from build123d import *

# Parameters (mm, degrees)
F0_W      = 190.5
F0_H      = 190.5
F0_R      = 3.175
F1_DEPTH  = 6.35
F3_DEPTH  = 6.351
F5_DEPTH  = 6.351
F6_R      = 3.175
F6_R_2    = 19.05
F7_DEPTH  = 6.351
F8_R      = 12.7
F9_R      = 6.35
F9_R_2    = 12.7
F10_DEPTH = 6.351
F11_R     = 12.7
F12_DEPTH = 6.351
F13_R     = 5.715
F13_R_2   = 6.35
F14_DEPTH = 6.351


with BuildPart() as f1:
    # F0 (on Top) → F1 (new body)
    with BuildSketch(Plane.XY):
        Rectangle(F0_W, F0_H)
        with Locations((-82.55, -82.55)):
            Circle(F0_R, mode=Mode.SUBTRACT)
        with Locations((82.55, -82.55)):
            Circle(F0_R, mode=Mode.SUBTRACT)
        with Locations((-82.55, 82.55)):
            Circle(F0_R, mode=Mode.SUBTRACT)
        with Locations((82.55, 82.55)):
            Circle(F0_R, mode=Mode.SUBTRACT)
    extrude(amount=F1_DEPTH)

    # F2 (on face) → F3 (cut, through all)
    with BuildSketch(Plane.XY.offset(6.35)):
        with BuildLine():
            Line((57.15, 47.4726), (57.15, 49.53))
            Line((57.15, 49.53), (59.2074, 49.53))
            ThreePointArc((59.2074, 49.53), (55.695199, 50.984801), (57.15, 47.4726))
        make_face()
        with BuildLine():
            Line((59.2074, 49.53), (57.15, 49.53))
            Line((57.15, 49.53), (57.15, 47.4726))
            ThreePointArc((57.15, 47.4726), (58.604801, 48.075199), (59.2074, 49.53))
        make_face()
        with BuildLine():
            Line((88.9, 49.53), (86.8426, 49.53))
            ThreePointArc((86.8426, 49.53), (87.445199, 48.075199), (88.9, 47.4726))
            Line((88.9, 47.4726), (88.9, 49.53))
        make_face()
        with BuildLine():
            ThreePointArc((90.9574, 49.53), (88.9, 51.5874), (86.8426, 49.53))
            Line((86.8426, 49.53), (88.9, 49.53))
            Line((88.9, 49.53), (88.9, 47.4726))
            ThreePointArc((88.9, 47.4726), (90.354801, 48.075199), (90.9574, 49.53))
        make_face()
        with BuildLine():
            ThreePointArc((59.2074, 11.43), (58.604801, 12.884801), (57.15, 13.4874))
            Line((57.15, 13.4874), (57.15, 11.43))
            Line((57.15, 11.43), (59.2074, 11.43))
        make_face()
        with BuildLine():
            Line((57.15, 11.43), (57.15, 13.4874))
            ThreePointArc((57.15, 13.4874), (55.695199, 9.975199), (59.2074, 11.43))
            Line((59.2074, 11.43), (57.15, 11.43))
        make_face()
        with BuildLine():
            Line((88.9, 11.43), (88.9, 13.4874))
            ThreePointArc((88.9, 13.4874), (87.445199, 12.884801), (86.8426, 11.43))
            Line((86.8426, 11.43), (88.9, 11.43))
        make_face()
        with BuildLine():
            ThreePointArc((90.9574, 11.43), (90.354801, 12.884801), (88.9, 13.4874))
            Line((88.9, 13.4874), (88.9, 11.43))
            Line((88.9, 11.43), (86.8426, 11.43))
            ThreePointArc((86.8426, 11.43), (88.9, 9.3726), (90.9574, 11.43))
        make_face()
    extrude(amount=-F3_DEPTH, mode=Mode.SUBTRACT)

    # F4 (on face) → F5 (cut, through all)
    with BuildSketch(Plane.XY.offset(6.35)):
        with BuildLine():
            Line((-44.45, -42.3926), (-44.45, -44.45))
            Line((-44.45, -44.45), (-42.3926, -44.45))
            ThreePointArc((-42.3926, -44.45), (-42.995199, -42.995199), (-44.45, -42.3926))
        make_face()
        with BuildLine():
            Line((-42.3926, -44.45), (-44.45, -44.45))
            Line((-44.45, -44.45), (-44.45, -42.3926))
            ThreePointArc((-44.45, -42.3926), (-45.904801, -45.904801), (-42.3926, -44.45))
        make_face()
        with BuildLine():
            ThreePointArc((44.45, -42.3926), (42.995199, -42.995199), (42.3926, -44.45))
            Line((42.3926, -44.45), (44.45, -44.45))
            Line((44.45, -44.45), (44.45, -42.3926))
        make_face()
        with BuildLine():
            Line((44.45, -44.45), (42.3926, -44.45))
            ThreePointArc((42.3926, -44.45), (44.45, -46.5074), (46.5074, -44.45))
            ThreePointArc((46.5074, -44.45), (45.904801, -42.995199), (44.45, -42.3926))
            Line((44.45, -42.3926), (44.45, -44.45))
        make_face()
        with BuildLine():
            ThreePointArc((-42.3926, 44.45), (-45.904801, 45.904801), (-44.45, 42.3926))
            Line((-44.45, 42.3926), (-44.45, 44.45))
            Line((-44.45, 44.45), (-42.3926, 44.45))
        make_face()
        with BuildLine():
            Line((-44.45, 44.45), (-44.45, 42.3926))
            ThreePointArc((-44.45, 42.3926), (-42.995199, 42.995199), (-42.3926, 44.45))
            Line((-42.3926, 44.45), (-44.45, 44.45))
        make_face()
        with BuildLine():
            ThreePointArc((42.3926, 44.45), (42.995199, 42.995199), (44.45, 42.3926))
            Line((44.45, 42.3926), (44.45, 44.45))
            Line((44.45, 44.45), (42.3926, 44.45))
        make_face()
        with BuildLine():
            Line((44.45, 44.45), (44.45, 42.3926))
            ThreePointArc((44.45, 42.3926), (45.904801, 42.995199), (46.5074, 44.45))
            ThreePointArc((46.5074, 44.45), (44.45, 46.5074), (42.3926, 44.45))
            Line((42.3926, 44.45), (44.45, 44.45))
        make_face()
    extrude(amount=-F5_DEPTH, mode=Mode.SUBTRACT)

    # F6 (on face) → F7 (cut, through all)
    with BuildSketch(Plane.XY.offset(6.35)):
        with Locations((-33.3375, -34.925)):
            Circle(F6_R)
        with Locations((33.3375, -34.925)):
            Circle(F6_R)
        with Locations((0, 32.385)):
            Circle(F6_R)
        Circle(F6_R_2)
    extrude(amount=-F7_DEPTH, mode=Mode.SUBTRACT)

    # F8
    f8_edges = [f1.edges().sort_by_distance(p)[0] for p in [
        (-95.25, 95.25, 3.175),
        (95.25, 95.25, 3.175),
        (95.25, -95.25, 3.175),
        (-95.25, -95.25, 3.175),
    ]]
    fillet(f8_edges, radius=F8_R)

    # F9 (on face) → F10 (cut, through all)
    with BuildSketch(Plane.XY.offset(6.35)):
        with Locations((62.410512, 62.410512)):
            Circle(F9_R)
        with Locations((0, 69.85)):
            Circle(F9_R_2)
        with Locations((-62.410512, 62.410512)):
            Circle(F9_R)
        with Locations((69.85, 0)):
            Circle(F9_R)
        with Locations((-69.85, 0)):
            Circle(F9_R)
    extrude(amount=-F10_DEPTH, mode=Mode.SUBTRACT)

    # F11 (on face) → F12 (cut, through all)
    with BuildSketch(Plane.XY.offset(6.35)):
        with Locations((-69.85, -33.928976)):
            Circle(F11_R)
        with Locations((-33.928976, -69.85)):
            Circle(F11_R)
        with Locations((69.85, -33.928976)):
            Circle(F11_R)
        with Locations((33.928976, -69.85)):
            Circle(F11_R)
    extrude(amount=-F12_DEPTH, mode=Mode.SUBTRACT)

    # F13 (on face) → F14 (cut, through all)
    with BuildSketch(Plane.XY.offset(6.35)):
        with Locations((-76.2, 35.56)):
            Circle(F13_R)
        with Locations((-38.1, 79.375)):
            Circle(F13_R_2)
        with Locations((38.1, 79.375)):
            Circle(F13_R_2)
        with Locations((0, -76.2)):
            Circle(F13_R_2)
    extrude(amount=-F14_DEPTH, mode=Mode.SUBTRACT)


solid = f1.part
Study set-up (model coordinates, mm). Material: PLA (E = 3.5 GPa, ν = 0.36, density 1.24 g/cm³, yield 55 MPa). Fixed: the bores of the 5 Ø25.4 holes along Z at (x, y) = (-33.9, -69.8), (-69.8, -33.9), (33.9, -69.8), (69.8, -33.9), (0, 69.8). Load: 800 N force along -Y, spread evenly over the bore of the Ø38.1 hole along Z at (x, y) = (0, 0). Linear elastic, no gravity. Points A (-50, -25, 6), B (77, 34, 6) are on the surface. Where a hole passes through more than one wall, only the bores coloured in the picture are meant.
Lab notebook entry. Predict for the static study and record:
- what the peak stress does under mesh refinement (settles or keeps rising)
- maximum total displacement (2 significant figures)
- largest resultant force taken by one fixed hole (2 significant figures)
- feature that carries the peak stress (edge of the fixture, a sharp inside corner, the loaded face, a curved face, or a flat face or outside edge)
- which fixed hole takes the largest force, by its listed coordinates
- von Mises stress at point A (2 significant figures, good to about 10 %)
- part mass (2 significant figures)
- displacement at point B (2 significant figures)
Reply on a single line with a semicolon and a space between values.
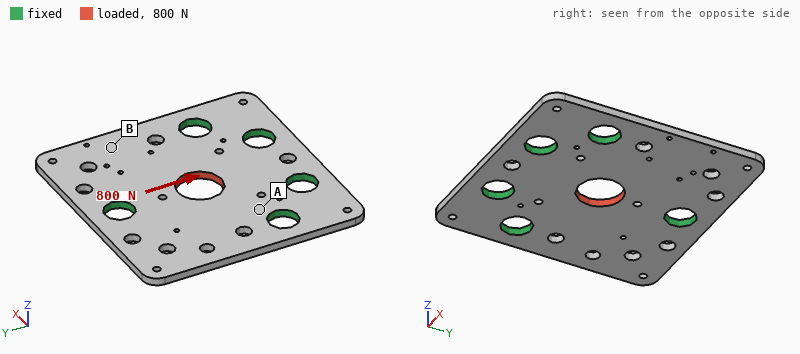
keeps rising; 14 µm; 270 N; a sharp inside corner; (0, 69.8); 0.41 MPa; 250 g; 4.0 µm
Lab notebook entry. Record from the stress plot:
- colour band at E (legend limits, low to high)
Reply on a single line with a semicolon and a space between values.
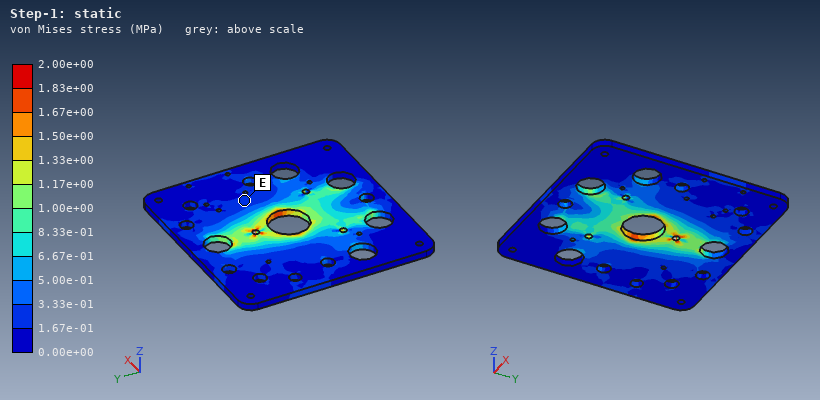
1.67e-01 to 3.33e-01 MPa
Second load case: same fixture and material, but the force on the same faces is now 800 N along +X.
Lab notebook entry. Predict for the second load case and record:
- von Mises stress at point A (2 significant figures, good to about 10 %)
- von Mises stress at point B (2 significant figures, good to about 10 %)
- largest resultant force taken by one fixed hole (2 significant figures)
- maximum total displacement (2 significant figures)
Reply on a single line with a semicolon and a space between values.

1.1 MPa; 0.25 MPa; 240 N; 20 µm
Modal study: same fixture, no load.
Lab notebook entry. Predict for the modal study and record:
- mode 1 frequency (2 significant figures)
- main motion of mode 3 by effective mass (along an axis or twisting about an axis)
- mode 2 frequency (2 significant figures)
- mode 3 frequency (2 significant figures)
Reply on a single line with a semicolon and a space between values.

350 Hz; along Z; 350 Hz; 900 Hz
